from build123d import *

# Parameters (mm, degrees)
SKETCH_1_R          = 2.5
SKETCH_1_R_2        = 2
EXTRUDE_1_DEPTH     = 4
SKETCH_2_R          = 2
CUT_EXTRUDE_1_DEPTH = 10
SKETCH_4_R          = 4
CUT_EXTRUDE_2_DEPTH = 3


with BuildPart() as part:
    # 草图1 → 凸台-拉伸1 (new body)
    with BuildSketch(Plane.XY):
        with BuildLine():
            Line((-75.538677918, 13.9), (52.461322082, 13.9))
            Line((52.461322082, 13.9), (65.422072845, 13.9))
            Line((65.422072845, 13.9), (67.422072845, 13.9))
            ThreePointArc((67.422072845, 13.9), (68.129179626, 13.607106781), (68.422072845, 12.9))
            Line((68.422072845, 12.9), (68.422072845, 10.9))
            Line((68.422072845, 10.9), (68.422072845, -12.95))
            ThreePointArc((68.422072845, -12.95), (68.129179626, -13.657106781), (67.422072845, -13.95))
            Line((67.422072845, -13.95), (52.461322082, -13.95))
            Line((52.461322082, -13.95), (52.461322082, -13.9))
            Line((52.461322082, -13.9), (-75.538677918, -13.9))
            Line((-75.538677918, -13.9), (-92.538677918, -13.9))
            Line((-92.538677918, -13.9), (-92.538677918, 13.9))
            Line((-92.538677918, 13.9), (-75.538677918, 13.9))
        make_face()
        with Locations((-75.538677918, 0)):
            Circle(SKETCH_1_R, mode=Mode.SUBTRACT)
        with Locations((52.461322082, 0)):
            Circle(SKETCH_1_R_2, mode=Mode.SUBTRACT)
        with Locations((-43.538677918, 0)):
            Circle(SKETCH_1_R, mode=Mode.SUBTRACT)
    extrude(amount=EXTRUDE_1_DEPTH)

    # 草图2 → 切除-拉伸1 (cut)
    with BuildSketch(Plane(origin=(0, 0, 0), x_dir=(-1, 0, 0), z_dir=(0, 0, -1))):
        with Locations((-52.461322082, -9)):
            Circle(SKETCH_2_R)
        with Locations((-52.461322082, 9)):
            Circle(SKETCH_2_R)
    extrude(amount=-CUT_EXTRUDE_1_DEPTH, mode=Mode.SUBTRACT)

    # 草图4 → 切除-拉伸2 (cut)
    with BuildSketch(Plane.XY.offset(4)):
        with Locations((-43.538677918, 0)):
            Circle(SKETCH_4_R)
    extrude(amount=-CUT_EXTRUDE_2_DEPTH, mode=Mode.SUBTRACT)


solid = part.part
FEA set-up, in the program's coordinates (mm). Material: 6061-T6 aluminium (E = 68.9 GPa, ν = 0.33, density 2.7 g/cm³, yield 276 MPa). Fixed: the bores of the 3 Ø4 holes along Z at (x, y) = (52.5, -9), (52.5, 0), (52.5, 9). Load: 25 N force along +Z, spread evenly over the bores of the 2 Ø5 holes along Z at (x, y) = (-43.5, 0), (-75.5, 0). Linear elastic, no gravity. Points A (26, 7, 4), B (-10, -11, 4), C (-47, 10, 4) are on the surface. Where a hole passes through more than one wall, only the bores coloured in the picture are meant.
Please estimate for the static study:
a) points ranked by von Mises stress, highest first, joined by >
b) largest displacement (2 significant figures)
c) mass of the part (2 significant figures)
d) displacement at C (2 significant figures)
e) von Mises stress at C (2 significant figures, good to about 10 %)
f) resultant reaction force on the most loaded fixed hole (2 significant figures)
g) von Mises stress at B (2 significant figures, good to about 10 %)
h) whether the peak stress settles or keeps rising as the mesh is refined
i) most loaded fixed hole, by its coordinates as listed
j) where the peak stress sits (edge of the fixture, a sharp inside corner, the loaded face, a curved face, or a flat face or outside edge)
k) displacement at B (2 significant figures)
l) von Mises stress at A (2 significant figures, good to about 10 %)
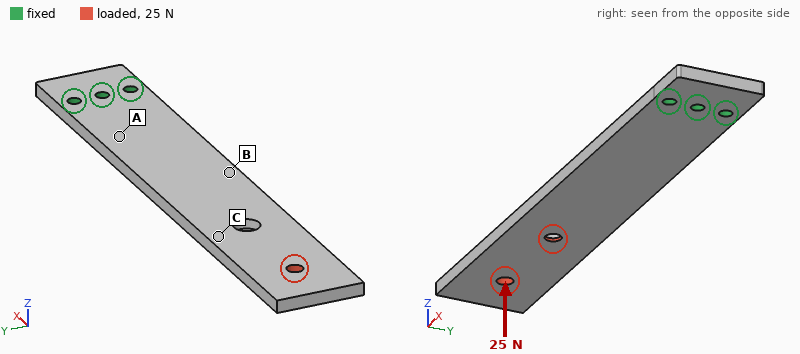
A > B > C
1.8 mm
47 g
1.0 mm
9.6 MPa
56 N
20 MPa
keeps rising
(52.5, 0)
edge of the fixture
0.44 mm
32 MPa
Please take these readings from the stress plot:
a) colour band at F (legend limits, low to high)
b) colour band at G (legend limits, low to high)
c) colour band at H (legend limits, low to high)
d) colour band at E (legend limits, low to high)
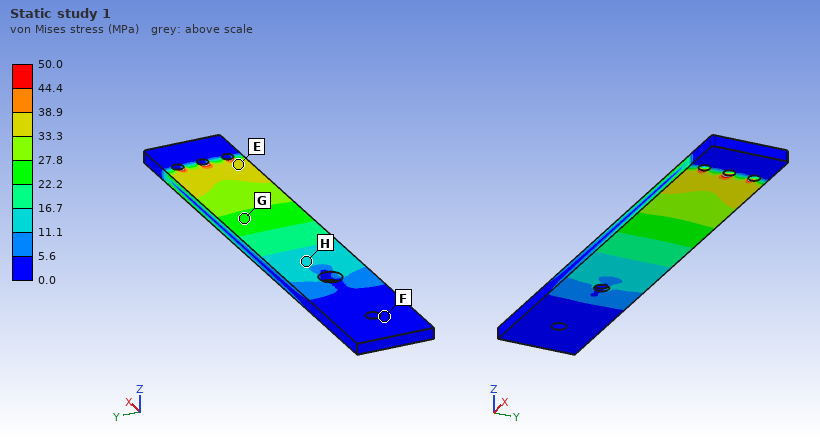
0.0 to 5.6 MPa
22.2 to 27.8 MPa
11.1 to 16.7 MPa
33.3 to 38.9 MPa
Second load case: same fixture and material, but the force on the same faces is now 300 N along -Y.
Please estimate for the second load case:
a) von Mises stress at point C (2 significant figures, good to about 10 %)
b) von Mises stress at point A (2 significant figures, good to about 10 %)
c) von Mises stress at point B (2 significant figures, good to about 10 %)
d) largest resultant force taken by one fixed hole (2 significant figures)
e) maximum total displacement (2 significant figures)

10.0 MPa
30 MPa
27 MPa
1.8 kN
0.49 mm
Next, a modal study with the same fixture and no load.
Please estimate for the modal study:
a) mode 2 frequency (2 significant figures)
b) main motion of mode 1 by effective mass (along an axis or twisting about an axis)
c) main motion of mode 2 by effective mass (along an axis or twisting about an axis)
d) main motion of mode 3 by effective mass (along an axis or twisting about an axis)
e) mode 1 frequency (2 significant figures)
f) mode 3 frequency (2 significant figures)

980 Hz
along Z
along Z
along Y
160 Hz
1100 Hz
